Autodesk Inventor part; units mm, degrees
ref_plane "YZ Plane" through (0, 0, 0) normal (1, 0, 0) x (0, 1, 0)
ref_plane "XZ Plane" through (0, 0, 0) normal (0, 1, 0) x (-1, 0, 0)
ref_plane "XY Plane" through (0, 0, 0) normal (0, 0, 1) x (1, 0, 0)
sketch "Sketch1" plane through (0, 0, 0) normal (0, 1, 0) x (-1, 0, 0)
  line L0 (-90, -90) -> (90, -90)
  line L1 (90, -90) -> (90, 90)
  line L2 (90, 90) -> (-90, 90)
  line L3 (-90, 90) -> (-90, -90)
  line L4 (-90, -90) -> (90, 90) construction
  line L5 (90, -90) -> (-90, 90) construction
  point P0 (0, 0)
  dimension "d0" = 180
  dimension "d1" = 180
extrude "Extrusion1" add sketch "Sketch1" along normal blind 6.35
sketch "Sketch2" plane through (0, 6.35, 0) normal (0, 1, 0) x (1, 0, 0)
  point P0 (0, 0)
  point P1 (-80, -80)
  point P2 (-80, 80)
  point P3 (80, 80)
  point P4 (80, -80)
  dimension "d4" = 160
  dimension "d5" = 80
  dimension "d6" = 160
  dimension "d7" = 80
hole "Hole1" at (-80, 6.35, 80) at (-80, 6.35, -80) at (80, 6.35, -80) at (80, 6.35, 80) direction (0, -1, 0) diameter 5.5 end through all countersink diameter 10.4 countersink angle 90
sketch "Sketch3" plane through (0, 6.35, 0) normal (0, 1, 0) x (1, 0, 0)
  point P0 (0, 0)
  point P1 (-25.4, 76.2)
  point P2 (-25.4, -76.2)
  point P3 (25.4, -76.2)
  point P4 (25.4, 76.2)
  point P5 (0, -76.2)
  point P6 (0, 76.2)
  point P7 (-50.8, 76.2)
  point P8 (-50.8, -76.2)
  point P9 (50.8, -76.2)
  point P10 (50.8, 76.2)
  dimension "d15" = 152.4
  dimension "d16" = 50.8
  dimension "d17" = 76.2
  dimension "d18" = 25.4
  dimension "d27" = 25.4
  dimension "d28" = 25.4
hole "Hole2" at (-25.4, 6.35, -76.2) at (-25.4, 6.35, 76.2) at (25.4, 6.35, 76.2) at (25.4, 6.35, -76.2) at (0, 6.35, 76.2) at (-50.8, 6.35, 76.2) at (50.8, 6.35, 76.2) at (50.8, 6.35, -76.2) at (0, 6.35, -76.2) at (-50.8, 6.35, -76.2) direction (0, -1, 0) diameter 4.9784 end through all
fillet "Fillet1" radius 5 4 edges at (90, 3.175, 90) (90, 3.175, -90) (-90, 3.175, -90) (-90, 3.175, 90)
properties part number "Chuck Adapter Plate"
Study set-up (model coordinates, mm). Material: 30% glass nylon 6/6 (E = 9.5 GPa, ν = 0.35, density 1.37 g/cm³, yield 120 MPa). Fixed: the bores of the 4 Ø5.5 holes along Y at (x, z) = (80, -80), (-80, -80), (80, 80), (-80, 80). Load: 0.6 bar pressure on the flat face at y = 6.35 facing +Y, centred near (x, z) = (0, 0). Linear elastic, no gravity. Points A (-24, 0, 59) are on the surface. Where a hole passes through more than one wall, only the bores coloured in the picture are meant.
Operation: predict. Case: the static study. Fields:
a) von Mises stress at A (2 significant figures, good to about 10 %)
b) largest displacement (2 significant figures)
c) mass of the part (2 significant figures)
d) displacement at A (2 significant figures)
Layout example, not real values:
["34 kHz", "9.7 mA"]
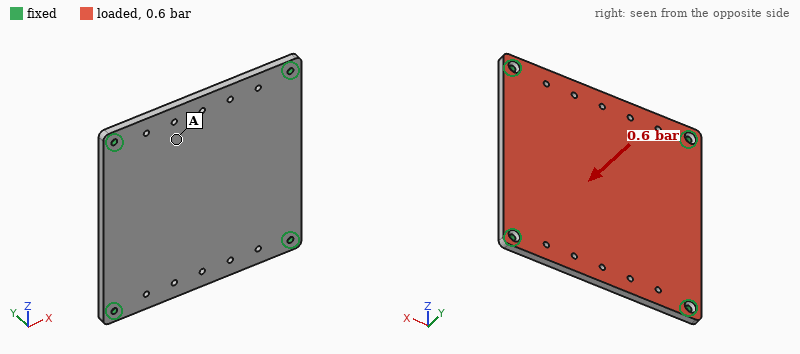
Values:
["12 MPa", "1.8 mm", "280 g", "1.2 mm"]
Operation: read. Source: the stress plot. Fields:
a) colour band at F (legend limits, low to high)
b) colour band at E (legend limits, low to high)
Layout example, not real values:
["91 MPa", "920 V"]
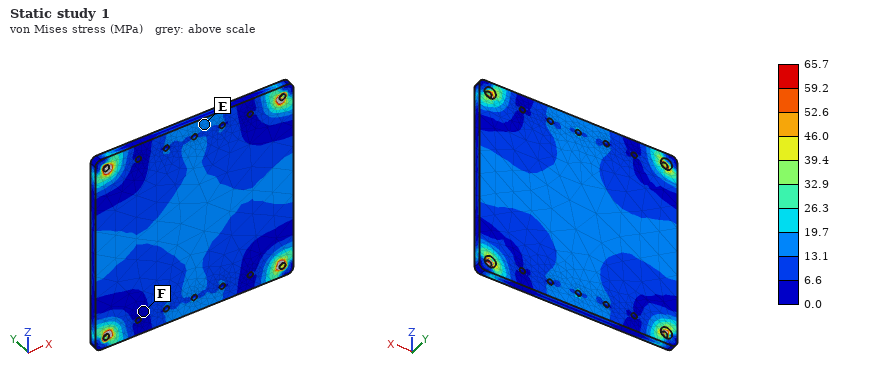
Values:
["0.0 to 6.6 MPa", "13.1 to 19.7 MPa"]
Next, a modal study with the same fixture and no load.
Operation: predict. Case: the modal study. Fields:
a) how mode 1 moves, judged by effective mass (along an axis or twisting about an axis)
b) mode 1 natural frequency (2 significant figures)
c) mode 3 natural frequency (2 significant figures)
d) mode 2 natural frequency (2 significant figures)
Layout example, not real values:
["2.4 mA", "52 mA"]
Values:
["along Y", "370 Hz", "670 Hz", "670 Hz"]
